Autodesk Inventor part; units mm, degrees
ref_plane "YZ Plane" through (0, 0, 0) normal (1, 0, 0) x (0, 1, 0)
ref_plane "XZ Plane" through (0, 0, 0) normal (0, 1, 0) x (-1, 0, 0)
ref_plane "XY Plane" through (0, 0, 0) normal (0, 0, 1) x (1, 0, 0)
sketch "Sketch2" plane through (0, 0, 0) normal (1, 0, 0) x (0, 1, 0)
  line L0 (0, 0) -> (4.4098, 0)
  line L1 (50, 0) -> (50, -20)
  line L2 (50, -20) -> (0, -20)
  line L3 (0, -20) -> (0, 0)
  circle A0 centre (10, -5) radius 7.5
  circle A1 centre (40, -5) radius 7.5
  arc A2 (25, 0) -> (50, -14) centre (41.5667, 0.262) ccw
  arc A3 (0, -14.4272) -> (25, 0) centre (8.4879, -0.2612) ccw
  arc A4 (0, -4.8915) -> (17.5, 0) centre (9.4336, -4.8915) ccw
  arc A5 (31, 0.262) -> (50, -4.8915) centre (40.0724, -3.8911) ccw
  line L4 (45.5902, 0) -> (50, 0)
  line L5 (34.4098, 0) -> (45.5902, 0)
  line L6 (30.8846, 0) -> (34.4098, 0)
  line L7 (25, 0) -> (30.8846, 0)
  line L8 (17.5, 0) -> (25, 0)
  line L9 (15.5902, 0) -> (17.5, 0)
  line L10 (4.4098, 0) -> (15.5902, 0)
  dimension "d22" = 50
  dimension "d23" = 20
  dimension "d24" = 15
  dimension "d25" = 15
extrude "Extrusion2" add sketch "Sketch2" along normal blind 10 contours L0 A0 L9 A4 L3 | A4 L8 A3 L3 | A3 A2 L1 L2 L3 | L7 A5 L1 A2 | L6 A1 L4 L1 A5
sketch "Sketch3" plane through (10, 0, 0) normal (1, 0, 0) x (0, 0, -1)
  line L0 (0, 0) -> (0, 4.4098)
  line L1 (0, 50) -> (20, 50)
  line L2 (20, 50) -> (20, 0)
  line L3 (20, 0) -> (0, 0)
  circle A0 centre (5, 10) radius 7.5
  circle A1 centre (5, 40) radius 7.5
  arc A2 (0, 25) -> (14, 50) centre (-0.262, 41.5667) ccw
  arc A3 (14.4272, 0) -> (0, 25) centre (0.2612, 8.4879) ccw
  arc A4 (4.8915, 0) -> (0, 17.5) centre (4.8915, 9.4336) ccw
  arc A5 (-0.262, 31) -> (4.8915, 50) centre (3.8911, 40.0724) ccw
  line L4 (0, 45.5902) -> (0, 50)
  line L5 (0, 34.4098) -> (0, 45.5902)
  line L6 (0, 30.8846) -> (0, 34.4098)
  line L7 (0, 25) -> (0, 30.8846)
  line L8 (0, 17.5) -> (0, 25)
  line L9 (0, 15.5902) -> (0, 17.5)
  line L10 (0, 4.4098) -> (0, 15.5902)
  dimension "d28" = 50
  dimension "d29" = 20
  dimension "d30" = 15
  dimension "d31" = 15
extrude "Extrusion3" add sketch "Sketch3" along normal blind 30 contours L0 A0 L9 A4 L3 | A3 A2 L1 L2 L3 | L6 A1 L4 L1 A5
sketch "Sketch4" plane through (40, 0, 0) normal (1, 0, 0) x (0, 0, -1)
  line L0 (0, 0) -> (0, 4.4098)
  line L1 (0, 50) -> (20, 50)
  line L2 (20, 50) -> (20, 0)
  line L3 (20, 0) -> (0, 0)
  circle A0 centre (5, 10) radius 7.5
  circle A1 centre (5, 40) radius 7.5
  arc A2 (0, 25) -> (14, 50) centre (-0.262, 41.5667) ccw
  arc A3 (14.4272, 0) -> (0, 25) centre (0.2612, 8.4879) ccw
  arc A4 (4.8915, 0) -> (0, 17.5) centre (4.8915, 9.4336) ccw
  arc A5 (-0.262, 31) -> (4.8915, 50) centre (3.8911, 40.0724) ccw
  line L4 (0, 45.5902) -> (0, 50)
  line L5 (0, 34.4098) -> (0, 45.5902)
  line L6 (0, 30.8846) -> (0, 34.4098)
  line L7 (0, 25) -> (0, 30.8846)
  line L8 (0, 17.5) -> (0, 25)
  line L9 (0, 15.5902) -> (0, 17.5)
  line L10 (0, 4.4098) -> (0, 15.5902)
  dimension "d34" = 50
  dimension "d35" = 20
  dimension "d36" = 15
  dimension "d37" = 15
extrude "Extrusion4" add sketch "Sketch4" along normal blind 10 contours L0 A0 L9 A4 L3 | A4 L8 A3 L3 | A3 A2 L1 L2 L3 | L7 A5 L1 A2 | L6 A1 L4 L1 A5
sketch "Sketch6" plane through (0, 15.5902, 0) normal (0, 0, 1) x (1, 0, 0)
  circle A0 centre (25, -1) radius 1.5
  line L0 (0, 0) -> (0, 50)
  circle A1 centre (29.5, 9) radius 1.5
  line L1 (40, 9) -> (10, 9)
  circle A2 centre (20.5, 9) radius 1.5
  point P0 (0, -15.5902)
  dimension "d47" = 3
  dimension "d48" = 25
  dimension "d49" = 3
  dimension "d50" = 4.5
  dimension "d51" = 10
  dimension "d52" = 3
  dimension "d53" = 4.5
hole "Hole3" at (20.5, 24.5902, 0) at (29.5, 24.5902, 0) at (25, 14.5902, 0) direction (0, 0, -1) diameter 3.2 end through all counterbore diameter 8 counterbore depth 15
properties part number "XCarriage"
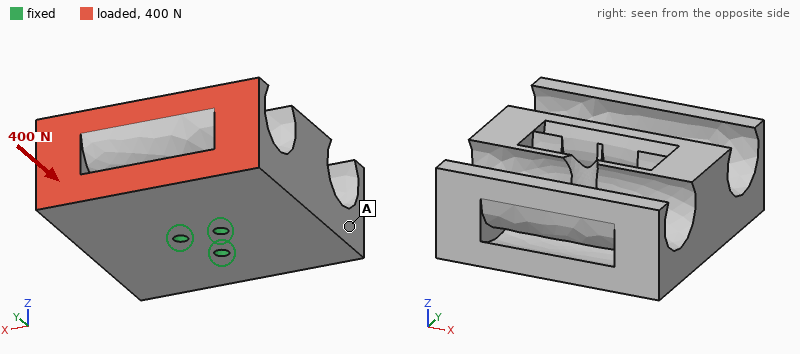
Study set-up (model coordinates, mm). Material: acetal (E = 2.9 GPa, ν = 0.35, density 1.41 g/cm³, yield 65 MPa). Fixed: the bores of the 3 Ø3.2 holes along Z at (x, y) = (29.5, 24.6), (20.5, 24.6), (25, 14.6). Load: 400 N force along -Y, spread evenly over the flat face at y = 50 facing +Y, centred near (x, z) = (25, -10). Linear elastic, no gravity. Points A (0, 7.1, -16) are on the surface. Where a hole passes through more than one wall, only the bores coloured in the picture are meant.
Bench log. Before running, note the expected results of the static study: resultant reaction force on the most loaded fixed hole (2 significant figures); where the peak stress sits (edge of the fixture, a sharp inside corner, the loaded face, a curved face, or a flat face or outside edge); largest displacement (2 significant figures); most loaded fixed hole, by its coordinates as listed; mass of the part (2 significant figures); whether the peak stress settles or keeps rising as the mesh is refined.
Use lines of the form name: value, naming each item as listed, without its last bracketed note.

resultant reaction force on the most loaded fixed hole: 190 N
where the peak stress sits: edge of the fixture
largest displacement: 0.78 mm
most loaded fixed hole, by its coordinates as listed: (25, 14.6)
mass of the part: 37 g
whether the peak stress settles or keeps rising as the mesh is refined: keeps rising
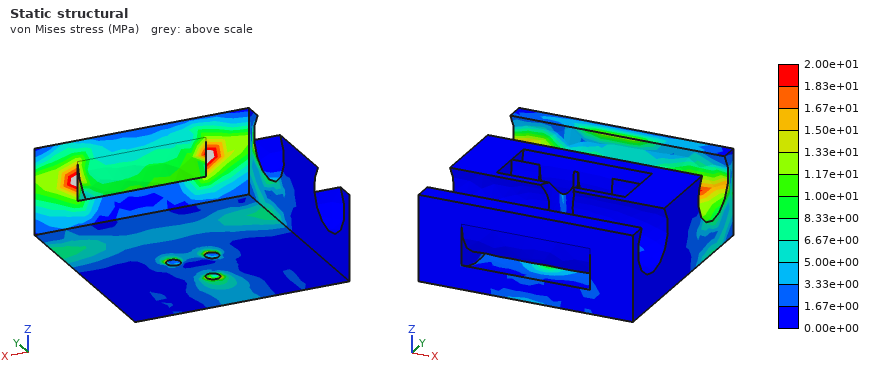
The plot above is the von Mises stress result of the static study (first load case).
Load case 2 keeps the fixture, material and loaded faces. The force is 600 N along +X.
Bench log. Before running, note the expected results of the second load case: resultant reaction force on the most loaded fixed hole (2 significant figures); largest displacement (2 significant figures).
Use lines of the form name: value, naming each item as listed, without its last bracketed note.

resultant reaction force on the most loaded fixed hole: 970 N
largest displacement: 0.60 mm
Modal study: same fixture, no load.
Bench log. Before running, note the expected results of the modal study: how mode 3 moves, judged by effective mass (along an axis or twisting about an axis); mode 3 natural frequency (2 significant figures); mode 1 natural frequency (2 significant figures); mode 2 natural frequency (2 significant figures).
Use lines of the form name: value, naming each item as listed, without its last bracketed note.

how mode 3 moves, judged by effective mass: twisting about Z
mode 3 natural frequency: 1900 Hz
mode 1 natural frequency: 1200 Hz
mode 2 natural frequency: 1200 Hz
